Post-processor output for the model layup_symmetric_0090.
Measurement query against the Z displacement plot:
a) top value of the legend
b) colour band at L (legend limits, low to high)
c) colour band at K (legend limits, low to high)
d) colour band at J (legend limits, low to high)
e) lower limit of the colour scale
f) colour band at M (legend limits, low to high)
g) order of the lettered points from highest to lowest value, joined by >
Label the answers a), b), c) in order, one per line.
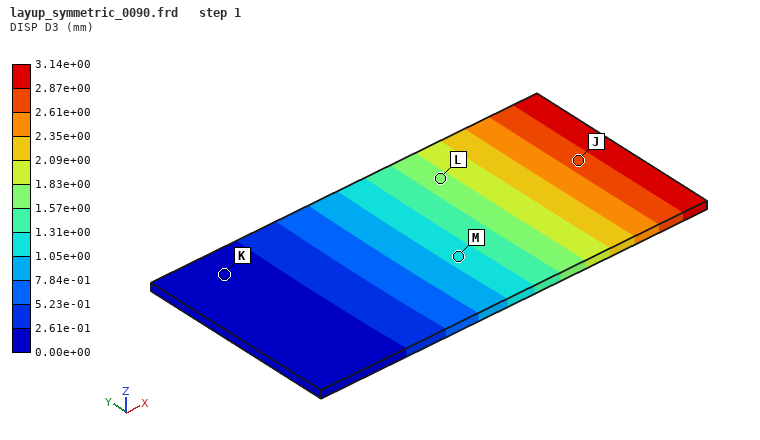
a) 3.14e+00 mm
b) 1.57e+00 to 1.83e+00 mm
c) 0.00e+00 to 2.61e-01 mm
d) 2.61e+00 to 2.87e+00 mm
e) 0.00e+00 mm
f) 1.05e+00 to 1.31e+00 mm
g) J > L > M > K
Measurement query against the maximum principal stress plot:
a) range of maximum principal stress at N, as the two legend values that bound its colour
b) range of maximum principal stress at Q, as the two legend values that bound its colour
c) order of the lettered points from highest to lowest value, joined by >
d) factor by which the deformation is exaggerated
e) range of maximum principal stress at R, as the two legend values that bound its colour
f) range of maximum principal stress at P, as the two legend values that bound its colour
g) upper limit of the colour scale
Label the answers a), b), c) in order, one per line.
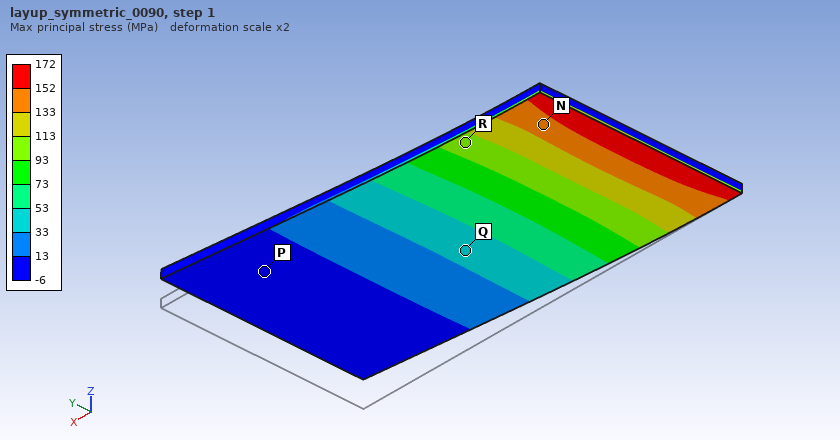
a) 133 to 152 MPa
b) 33 to 53 MPa
c) N > R > Q > P
d) 2
e) 93 to 113 MPa
f) -6 to 13 MPa
g) 172 MPa
